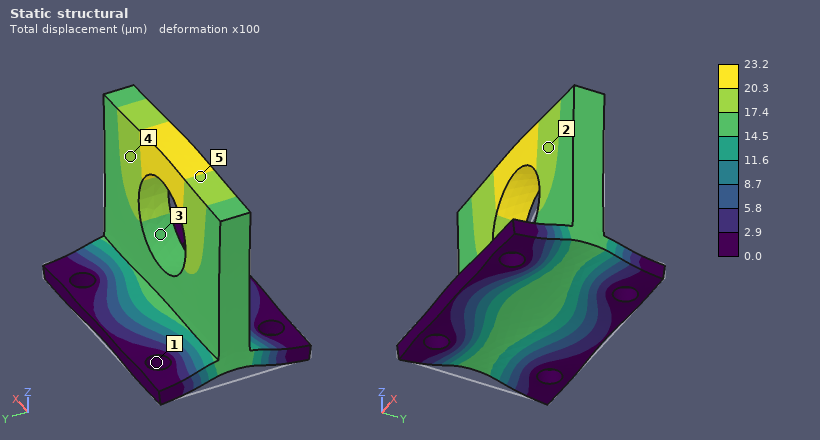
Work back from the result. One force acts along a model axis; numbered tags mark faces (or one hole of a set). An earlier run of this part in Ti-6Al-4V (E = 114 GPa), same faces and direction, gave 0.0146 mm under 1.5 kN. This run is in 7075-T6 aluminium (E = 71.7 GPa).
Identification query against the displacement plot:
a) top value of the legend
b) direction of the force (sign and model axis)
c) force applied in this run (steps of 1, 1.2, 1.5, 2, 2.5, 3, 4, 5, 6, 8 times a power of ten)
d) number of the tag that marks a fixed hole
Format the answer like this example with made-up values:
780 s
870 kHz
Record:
23.2 µm
+Z
1.5 kN
1
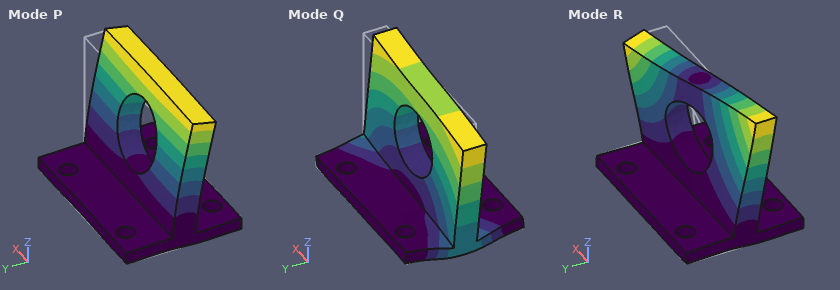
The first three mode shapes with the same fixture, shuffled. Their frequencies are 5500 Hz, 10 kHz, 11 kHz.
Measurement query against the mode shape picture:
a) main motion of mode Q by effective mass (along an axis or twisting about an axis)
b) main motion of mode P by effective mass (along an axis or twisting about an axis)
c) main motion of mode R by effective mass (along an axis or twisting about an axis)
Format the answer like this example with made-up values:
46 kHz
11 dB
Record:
along X
along Y
twisting about Z
